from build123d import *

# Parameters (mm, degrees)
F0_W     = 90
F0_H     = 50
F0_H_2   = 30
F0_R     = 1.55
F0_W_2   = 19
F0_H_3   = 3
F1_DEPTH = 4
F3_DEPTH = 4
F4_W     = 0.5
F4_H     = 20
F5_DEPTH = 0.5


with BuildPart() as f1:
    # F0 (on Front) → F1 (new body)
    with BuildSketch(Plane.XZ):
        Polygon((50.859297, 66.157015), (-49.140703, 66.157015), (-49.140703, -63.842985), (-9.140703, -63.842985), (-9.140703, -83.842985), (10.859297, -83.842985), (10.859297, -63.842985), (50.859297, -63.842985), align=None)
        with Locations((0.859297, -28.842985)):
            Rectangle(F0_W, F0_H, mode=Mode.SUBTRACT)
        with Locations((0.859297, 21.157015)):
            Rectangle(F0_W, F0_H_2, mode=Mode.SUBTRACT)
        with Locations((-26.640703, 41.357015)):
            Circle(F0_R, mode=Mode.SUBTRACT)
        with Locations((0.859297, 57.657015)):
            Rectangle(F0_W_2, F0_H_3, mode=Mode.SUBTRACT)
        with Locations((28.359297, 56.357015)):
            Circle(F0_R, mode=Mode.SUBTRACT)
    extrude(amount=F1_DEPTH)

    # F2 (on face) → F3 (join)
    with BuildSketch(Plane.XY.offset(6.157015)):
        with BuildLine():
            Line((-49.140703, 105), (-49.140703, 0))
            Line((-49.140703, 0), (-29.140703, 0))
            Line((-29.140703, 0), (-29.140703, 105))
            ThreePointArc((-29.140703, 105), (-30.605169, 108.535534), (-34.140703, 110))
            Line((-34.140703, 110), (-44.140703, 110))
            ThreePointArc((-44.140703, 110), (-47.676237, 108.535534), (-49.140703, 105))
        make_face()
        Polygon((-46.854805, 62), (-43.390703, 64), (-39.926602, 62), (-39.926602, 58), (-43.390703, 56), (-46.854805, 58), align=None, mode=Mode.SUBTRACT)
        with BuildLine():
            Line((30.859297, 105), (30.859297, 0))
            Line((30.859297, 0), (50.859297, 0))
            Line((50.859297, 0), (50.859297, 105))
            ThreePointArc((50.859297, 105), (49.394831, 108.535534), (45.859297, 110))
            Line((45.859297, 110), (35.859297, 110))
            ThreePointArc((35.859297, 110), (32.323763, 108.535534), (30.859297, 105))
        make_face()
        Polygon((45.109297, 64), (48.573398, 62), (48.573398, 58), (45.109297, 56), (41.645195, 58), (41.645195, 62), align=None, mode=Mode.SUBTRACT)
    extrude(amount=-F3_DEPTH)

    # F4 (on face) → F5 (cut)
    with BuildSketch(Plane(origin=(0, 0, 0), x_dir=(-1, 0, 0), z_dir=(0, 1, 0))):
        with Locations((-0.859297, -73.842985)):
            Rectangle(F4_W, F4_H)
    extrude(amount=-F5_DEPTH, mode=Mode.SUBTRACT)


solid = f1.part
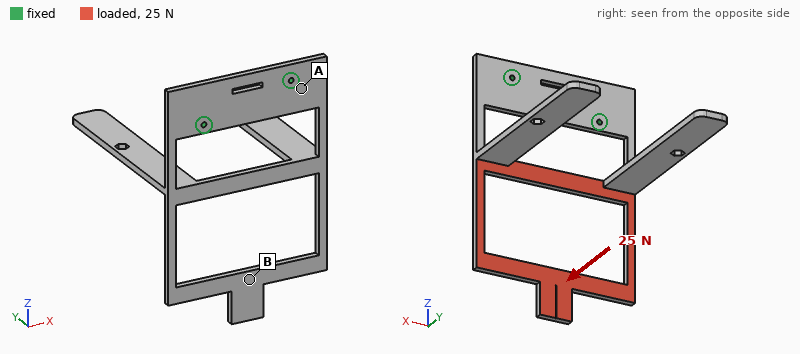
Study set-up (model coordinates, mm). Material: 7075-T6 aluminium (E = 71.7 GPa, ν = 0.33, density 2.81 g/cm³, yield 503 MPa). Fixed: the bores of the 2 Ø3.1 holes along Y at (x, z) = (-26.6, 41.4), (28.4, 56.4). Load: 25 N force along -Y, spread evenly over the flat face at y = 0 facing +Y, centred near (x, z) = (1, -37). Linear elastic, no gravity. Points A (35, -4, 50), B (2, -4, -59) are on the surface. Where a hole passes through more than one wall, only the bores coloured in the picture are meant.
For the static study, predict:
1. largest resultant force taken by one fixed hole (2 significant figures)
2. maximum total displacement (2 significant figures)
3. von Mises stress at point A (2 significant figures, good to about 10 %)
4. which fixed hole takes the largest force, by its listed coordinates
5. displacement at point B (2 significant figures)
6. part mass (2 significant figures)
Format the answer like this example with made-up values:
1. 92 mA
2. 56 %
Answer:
1. 16 N
2. 2.3 mm
3. 13 MPa
4. (28.4, 56.4)
5. 1.7 mm
6. 120 g
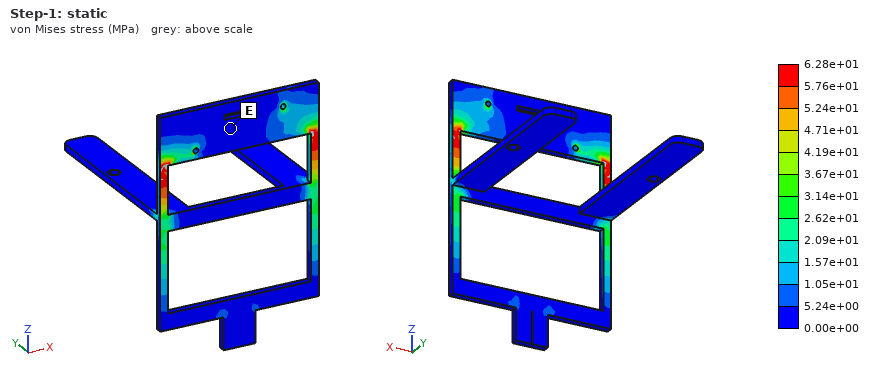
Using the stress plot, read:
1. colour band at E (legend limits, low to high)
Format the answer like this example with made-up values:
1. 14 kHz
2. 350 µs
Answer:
1. 0.00e+00 to 5.24e+00 MPa
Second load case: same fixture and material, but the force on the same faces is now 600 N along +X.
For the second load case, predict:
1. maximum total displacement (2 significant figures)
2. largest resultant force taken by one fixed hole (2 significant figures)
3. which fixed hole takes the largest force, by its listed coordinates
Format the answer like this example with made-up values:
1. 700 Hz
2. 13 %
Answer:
1. 1.7 mm
2. 1.2 kN
3. (-26.6, 41.4)
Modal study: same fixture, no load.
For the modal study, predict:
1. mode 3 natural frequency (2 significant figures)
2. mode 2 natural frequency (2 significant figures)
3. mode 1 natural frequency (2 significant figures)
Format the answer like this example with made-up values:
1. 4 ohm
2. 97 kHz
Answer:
1. 200 Hz
2. 160 Hz
3. 77 Hz
